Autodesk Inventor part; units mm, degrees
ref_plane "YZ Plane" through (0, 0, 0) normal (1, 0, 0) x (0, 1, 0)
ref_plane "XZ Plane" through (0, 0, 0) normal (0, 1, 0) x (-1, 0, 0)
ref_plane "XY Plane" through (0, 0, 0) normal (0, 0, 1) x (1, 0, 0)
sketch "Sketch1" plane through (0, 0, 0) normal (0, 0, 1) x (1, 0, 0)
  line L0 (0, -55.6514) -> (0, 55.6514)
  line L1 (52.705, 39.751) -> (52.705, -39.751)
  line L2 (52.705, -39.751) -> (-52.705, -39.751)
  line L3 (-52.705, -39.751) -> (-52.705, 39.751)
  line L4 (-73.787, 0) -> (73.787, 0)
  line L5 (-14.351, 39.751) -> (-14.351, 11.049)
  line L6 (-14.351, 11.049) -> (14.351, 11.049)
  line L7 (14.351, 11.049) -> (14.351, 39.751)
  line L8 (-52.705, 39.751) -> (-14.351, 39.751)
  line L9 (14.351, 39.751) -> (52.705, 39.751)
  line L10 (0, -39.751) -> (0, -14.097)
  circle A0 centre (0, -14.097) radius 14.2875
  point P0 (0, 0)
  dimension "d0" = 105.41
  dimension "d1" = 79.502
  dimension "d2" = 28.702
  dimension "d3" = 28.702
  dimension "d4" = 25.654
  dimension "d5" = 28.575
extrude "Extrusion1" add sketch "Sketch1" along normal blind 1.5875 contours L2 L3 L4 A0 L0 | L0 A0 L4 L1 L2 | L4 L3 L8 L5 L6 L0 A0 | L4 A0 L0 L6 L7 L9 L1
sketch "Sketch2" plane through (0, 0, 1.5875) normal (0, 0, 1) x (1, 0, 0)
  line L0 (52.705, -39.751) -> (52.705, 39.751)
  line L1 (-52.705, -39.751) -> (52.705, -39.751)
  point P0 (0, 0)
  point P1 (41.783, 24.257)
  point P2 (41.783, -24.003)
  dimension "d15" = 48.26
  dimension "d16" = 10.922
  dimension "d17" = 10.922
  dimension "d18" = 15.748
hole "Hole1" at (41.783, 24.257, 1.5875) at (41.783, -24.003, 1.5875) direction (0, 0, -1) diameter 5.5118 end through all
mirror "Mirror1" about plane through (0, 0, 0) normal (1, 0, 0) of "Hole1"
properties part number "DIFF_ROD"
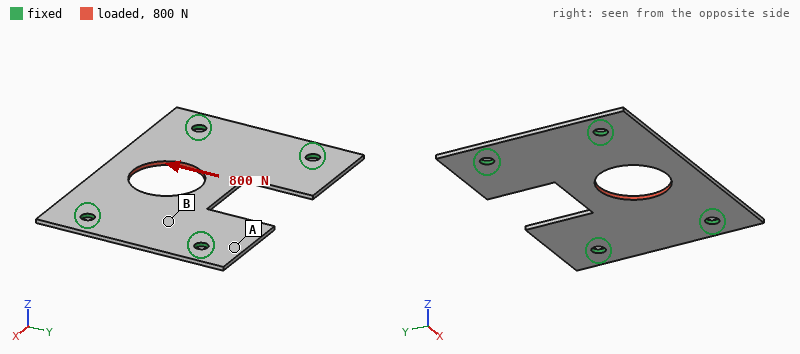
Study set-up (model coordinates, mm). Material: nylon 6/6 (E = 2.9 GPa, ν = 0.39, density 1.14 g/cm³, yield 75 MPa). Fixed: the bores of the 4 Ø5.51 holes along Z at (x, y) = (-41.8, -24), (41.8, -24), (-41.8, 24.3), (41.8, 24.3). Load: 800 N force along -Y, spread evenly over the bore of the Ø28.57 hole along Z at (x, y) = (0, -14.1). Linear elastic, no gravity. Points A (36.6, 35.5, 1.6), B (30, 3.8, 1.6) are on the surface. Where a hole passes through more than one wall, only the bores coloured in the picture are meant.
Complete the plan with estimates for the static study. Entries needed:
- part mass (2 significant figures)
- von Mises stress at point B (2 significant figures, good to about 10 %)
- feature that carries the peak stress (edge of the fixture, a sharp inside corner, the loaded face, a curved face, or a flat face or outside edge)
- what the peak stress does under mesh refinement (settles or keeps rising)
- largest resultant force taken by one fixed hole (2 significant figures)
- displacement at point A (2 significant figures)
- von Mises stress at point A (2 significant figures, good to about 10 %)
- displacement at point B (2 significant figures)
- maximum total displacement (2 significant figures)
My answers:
12 g
6.9 MPa
edge of the fixture
keeps rising
270 N
0.046 mm
2.2 MPa
0.060 mm
0.27 mm
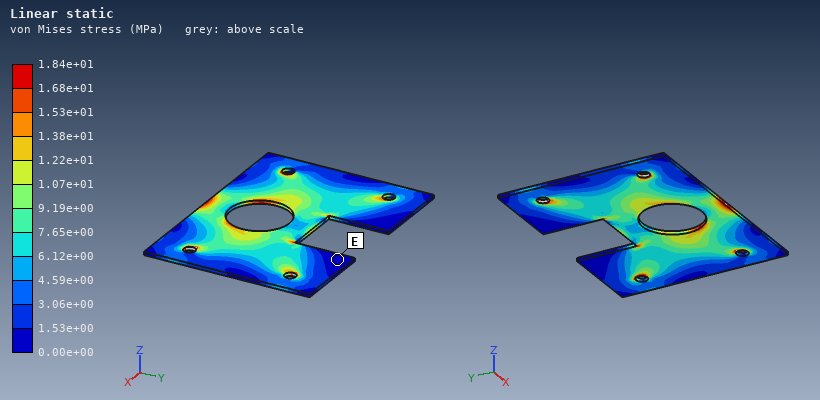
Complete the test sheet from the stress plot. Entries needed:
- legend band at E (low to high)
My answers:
0.00e+00 to 1.53e+00 MPa
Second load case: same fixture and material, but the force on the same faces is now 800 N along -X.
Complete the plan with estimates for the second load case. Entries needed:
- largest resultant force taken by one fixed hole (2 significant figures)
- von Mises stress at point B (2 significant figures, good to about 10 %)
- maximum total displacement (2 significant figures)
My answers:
300 N
2.6 MPa
99 µm
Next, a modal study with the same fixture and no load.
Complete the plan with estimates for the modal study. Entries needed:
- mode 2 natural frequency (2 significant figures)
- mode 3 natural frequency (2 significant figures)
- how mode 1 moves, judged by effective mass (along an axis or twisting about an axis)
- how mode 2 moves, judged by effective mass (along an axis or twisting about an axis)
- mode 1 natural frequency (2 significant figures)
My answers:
530 Hz
750 Hz
along Z
twisting about X
420 Hz
